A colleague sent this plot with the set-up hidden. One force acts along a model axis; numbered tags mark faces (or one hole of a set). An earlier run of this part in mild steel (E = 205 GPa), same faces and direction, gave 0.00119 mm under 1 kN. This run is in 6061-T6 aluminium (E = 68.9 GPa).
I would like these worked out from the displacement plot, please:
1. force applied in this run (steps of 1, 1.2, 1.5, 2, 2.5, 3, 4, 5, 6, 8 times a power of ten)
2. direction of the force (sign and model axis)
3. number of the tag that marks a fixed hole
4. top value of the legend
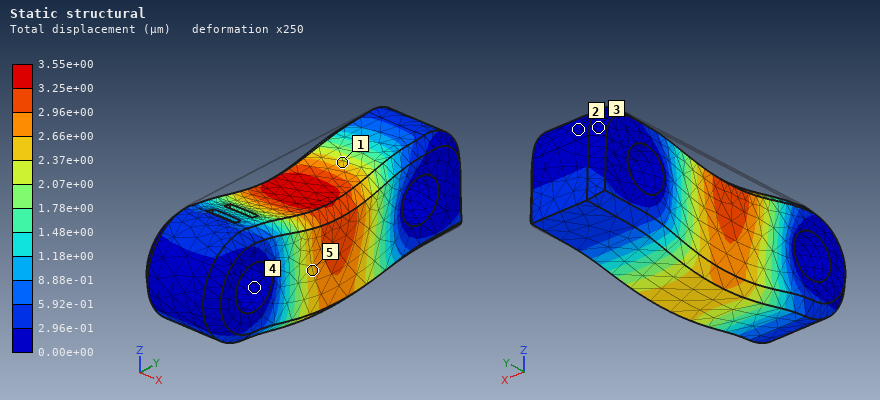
1 kN
-Z
4
3.55e+00 µm
